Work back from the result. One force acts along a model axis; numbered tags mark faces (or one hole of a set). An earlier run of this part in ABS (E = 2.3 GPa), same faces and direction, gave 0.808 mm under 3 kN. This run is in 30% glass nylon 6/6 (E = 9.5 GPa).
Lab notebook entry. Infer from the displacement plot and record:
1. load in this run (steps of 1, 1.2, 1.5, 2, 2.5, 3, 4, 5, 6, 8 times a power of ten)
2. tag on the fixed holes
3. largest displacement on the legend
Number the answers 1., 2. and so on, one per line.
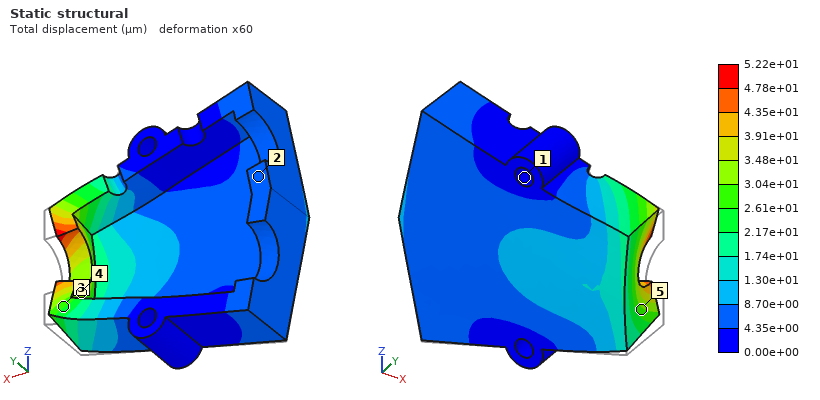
1. 800 N
2. 1
3. 5.22e+01 µm
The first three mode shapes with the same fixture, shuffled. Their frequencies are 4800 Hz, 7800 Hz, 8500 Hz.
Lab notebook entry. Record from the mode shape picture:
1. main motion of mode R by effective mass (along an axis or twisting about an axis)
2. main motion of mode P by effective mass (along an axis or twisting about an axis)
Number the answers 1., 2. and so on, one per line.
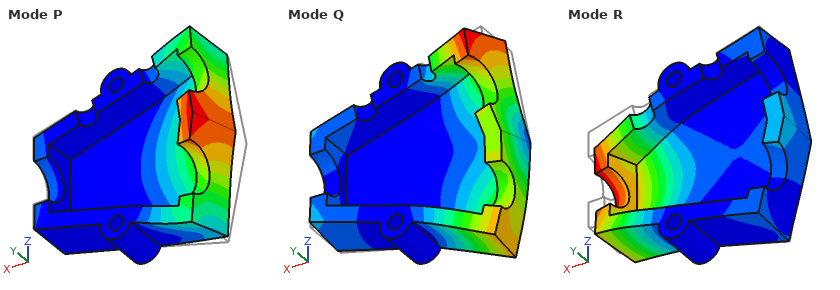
1. along Y
2. along Y
